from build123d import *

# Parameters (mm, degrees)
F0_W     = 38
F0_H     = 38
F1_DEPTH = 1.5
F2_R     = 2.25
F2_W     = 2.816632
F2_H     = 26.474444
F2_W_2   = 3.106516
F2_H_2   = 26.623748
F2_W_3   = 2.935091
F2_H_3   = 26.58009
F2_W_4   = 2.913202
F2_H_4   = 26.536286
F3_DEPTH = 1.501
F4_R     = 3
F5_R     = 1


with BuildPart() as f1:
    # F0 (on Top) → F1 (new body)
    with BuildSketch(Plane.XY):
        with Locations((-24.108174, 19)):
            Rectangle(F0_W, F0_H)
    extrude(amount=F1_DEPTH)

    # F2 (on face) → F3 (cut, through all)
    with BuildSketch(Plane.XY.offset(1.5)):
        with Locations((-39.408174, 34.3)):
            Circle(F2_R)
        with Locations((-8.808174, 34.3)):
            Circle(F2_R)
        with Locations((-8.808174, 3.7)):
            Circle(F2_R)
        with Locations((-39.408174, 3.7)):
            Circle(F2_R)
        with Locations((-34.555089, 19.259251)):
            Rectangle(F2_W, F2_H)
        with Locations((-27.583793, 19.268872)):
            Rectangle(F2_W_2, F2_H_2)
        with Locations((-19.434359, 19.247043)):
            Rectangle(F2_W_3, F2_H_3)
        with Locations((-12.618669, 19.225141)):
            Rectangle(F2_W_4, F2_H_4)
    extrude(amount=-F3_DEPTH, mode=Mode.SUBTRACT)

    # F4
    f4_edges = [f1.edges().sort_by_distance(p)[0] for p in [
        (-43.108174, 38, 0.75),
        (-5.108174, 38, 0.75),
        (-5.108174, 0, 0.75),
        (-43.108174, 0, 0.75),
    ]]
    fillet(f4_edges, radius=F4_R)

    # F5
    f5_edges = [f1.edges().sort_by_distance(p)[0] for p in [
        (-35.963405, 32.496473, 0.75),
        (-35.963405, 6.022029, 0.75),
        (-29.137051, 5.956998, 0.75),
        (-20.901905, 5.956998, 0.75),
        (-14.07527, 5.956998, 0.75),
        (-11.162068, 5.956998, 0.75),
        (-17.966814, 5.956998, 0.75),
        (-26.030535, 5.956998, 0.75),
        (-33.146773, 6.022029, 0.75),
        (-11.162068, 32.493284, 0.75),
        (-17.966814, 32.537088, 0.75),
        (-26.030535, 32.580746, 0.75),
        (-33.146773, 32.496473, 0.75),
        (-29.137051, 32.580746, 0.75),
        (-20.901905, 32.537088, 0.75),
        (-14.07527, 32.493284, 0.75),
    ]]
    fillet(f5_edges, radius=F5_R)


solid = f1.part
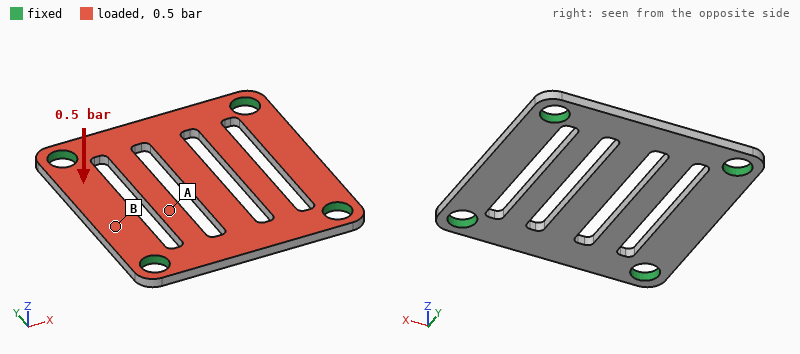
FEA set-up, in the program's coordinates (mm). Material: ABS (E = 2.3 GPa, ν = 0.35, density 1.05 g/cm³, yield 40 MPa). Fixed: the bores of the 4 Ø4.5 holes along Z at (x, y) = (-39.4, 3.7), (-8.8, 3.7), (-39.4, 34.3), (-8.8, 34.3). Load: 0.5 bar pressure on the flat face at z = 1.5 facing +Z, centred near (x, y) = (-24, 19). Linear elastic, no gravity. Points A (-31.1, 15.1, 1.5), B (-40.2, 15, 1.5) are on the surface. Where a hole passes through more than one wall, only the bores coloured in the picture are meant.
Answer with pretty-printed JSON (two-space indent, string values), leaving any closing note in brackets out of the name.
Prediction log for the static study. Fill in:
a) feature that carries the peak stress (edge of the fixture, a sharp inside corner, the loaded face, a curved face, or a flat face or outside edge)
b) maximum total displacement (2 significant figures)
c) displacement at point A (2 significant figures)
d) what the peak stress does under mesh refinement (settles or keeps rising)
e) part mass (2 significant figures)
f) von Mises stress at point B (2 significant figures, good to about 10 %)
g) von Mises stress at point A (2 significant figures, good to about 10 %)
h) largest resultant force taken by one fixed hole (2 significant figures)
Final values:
{
  "feature that carries the peak stress": "edge of the fixture",
  "maximum total displacement": "0.64 mm",
  "displacement at point A": "0.39 mm",
  "what the peak stress does under mesh refinement": "keeps rising",
  "part mass": "1.7 g",
  "von Mises stress at point B": "2.6 MPa",
  "von Mises stress at point A": "5.7 MPa",
  "largest resultant force taken by one fixed hole": "14 N"
}
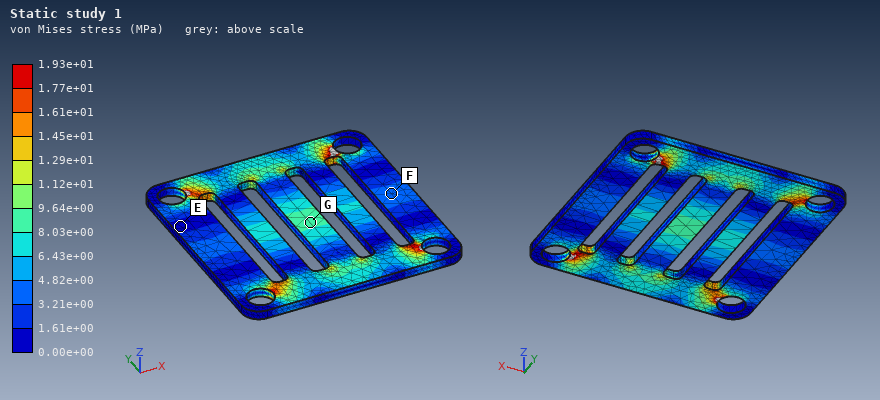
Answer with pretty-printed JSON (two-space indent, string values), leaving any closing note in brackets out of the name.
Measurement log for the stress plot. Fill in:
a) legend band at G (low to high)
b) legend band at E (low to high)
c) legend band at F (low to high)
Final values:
{
  "legend band at G": "8.03e+00 to 9.64e+00 MPa",
  "legend band at E": "0.00e+00 to 1.61e+00 MPa",
  "legend band at F": "3.21e+00 to 4.82e+00 MPa"
}
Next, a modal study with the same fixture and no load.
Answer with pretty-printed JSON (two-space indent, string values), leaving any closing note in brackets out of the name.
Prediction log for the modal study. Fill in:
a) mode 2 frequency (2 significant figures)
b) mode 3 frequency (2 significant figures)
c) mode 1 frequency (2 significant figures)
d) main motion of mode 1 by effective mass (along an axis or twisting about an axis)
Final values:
{
  "mode 2 frequency": "2200 Hz",
  "mode 3 frequency": "2300 Hz",
  "mode 1 frequency": "1400 Hz",
  "main motion of mode 1 by effective mass": "along Z"
}
